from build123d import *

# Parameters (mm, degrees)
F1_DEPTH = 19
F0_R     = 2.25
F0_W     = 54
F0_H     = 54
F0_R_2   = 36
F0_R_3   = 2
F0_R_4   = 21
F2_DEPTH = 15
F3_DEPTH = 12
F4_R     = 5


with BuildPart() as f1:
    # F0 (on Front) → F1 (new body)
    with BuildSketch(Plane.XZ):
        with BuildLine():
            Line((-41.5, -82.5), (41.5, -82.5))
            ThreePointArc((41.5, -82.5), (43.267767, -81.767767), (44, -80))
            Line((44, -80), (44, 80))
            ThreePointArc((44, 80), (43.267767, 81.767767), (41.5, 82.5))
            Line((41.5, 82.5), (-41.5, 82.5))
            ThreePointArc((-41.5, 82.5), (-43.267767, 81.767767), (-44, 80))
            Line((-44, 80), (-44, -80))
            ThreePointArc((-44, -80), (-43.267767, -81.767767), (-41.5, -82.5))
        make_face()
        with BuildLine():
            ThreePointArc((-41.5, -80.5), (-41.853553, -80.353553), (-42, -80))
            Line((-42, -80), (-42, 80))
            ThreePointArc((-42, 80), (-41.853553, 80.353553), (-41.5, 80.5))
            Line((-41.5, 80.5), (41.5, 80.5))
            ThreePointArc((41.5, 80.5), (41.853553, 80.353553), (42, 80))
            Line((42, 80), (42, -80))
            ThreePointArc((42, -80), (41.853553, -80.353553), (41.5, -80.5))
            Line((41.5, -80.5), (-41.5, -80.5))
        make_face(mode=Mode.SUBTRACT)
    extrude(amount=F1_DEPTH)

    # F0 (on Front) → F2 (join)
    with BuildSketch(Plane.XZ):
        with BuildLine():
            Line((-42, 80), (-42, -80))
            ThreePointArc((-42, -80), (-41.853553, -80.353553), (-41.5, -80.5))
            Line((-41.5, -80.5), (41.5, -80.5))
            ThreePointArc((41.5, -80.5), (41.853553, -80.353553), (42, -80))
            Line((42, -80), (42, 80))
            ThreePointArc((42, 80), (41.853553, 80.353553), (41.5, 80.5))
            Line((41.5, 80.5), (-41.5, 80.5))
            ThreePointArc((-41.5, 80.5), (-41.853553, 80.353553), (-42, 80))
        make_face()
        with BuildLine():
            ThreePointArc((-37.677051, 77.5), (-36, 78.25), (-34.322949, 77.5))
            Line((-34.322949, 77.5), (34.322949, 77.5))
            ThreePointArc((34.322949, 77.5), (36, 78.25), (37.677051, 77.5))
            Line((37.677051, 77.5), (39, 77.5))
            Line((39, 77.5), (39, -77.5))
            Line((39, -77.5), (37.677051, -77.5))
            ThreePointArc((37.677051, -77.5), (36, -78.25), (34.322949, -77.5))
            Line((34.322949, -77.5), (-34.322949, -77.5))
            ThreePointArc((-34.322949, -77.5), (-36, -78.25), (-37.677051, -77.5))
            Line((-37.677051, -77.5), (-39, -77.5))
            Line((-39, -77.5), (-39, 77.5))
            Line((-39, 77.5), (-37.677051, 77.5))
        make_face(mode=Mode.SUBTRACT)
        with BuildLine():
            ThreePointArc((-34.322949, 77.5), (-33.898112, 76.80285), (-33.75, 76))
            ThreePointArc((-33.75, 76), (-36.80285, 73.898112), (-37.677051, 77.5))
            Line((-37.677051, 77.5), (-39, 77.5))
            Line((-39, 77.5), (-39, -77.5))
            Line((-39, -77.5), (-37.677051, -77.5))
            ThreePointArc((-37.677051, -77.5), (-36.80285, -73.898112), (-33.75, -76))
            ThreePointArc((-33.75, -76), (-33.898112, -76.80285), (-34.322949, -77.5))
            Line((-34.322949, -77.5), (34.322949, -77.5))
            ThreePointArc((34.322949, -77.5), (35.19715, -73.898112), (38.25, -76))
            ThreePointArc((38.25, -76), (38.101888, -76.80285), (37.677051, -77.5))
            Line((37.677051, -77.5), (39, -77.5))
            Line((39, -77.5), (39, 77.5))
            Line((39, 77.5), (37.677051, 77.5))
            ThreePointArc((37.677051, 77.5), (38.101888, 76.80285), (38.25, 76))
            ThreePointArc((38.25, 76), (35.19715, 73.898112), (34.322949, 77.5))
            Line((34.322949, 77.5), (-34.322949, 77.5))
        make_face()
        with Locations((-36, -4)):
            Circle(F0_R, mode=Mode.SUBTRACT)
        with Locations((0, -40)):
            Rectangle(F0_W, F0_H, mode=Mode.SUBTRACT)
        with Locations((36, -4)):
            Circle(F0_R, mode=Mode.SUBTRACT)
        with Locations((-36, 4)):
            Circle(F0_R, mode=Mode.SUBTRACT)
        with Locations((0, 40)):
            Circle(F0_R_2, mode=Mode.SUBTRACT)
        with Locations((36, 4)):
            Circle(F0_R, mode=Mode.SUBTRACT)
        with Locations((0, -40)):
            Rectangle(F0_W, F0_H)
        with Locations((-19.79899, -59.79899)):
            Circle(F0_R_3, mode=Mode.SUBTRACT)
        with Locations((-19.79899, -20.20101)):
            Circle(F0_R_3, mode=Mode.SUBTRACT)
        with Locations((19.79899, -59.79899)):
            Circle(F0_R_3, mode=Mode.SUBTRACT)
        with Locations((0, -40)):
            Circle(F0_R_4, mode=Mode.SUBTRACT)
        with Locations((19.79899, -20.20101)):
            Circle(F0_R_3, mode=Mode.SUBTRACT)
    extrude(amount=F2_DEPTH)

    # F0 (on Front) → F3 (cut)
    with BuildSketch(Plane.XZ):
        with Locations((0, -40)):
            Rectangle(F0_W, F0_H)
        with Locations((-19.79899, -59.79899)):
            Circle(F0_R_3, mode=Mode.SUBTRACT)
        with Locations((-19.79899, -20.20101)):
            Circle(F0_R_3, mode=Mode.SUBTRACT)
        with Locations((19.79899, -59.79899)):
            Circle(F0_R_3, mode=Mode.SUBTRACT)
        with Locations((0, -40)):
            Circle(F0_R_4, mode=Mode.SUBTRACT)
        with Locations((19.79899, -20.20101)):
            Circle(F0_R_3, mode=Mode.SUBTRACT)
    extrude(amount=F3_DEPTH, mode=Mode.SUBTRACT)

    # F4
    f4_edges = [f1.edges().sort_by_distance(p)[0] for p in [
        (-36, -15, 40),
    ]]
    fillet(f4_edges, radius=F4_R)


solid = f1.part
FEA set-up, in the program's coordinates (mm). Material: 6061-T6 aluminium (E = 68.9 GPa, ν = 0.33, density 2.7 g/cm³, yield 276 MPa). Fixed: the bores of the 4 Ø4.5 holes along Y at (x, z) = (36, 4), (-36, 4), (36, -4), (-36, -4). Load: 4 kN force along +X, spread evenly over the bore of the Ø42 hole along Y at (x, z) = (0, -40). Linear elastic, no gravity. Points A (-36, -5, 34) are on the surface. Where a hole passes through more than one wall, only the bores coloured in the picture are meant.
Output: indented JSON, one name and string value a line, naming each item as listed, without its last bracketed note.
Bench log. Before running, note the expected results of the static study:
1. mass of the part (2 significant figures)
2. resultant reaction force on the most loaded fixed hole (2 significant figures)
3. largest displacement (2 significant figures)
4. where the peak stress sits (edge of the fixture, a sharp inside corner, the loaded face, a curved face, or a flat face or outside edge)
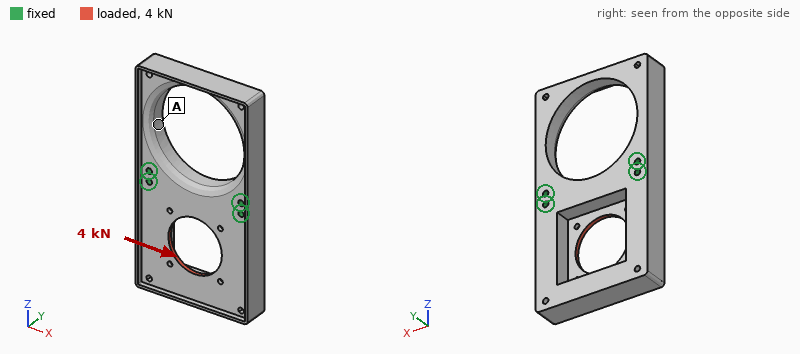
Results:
{
  "mass of the part": "320 g",
  "resultant reaction force on the most loaded fixed hole": "2.5 kN",
  "largest displacement": "49 µm",
  "where the peak stress sits": "a curved face"
}
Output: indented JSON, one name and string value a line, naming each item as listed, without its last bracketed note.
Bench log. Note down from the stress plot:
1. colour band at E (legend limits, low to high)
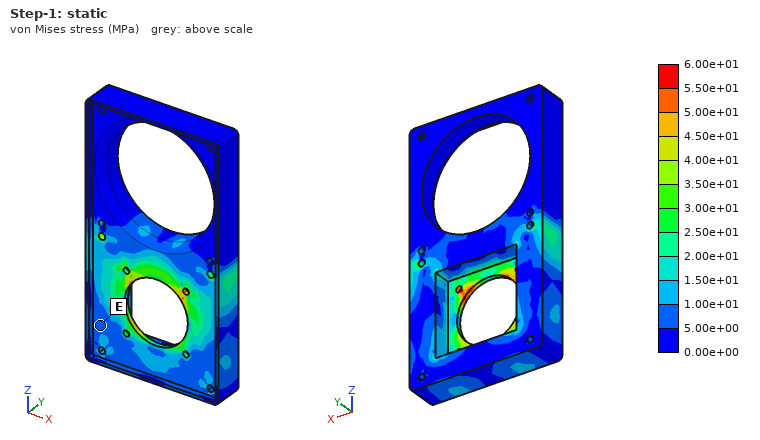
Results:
{
  "colour band at E": "5.00e+00 to 1.00e+01 MPa"
}
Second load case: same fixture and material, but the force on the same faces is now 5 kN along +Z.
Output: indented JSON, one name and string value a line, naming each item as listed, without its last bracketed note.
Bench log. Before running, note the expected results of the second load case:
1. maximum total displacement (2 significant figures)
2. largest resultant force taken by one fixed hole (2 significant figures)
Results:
{
  "maximum total displacement": "65 µm",
  "largest resultant force taken by one fixed hole": "1.7 kN"
}
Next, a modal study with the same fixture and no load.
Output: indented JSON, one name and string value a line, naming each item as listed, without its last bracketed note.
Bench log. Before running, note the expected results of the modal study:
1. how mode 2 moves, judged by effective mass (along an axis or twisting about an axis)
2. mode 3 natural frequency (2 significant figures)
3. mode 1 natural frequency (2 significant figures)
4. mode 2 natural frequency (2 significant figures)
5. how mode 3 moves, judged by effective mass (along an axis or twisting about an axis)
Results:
{
  "how mode 2 moves, judged by effective mass": "along Y",
  "mode 3 natural frequency": "2100 Hz",
  "mode 1 natural frequency": "1400 Hz",
  "mode 2 natural frequency": "1500 Hz",
  "how mode 3 moves, judged by effective mass": "along X"
}
